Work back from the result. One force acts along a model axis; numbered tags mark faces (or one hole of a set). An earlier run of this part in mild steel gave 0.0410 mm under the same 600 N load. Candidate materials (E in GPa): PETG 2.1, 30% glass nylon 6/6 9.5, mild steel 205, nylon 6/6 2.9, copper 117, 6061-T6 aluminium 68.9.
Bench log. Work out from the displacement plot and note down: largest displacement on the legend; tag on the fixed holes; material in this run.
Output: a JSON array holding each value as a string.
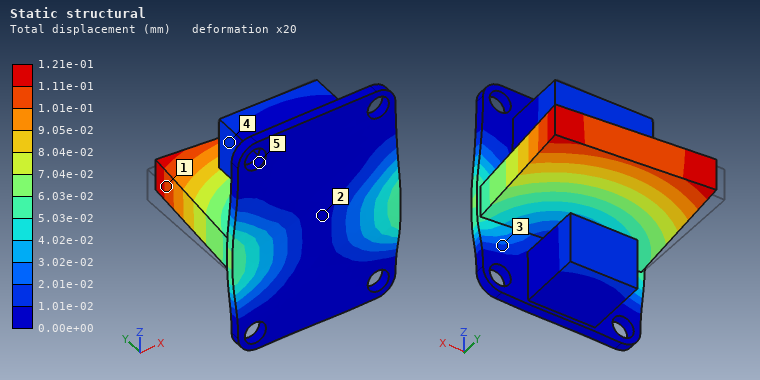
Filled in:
["1.21e-01 mm", "5", "6061-T6 aluminium"]
